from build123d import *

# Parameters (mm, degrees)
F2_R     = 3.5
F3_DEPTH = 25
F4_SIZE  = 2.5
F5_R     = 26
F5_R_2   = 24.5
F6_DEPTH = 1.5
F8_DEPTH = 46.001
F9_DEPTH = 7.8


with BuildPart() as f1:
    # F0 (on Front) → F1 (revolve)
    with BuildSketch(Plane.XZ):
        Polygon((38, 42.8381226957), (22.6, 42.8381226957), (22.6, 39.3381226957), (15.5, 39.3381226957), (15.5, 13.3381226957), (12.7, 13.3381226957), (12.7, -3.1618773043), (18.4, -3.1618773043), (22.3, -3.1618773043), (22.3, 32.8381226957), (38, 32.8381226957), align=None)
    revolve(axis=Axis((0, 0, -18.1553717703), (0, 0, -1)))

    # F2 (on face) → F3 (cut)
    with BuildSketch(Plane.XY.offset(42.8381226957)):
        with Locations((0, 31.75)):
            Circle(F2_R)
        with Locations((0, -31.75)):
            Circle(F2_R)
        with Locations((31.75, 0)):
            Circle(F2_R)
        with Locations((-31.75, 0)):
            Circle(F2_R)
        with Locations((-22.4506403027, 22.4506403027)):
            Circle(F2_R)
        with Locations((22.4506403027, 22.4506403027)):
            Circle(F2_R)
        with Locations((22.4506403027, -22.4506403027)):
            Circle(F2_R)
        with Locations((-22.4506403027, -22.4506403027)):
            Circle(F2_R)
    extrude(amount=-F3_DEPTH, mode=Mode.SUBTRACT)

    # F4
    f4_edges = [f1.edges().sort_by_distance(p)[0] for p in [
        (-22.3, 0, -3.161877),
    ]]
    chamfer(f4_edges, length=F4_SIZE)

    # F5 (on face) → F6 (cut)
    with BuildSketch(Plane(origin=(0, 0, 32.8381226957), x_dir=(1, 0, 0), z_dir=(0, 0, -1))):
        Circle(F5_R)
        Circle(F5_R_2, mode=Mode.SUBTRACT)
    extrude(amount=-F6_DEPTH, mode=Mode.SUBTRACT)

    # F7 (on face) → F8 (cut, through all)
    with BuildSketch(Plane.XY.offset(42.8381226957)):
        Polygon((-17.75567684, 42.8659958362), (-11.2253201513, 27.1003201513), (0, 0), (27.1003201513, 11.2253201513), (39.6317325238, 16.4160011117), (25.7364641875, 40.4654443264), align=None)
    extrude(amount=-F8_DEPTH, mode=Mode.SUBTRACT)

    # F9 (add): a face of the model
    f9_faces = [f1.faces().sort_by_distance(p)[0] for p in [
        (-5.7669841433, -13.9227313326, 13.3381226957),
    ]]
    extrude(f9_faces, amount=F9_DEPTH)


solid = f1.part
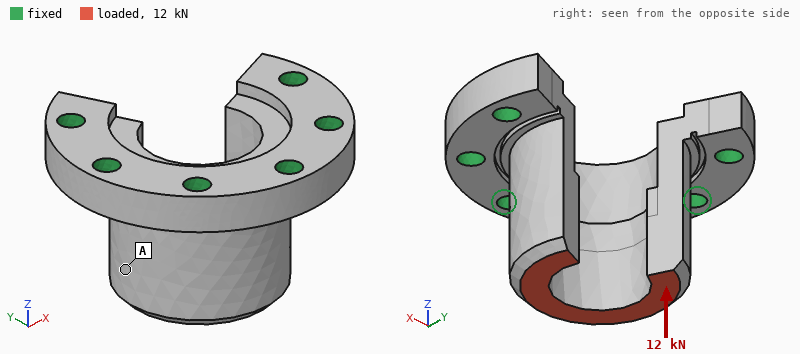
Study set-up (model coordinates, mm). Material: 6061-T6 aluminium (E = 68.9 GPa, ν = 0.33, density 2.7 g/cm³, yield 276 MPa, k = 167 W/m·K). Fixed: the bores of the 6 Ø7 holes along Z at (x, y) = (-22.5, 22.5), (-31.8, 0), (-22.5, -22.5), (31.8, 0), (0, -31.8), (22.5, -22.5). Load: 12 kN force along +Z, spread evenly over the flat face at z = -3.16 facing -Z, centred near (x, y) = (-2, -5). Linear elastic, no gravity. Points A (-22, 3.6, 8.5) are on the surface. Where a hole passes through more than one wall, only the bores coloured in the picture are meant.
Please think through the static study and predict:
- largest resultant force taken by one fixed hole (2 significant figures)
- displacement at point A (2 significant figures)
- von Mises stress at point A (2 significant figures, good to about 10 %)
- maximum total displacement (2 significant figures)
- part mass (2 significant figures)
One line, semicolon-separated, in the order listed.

2.6 kN; 22 µm; 15 MPa; 39 µm; 130 g
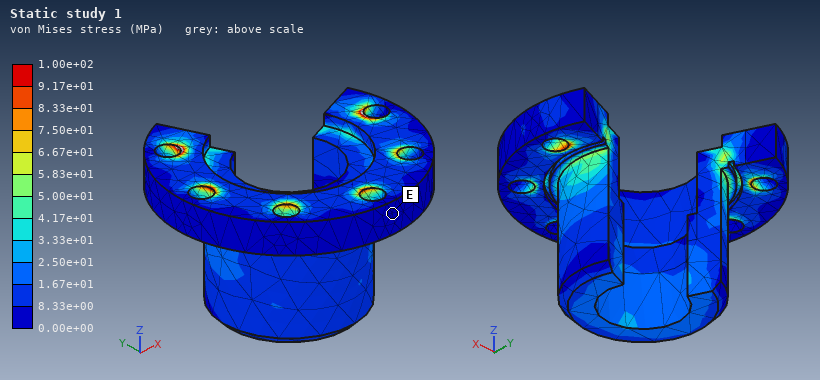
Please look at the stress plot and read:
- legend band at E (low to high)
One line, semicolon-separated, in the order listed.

0.00e+00 to 8.33e+00 MPa
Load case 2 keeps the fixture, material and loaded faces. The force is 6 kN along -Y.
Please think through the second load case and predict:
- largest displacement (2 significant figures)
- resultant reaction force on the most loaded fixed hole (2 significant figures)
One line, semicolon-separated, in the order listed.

0.14 mm; 4.0 kN
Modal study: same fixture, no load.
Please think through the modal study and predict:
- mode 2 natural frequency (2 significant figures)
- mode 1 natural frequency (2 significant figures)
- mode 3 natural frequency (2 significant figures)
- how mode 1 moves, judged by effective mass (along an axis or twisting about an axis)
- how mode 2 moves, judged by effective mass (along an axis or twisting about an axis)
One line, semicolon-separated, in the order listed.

7500 Hz; 5700 Hz; 8900 Hz; along X; along Y
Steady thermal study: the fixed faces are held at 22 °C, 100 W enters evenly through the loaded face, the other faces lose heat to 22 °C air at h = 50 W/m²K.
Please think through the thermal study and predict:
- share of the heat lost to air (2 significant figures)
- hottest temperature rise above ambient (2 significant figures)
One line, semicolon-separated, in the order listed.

9.1 %; 39 K
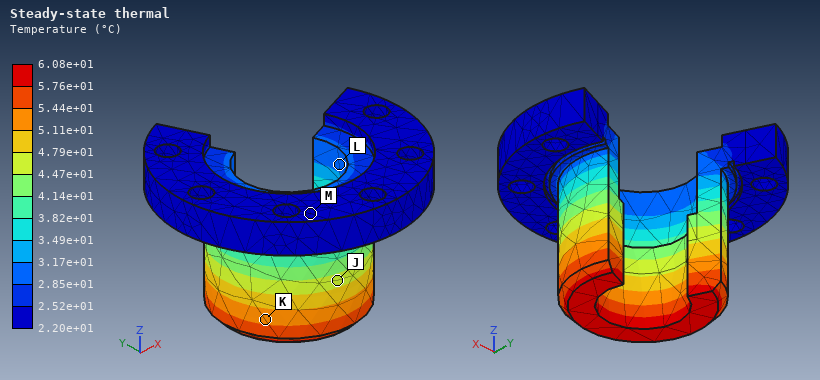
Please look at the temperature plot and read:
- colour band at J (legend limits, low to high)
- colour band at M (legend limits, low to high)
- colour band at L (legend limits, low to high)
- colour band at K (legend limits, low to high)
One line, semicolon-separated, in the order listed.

4.47e+01 to 4.79e+01 °C; 2.20e+01 to 2.52e+01 °C; 2.85e+01 to 3.17e+01 °C; 5.11e+01 to 5.44e+01 °C
